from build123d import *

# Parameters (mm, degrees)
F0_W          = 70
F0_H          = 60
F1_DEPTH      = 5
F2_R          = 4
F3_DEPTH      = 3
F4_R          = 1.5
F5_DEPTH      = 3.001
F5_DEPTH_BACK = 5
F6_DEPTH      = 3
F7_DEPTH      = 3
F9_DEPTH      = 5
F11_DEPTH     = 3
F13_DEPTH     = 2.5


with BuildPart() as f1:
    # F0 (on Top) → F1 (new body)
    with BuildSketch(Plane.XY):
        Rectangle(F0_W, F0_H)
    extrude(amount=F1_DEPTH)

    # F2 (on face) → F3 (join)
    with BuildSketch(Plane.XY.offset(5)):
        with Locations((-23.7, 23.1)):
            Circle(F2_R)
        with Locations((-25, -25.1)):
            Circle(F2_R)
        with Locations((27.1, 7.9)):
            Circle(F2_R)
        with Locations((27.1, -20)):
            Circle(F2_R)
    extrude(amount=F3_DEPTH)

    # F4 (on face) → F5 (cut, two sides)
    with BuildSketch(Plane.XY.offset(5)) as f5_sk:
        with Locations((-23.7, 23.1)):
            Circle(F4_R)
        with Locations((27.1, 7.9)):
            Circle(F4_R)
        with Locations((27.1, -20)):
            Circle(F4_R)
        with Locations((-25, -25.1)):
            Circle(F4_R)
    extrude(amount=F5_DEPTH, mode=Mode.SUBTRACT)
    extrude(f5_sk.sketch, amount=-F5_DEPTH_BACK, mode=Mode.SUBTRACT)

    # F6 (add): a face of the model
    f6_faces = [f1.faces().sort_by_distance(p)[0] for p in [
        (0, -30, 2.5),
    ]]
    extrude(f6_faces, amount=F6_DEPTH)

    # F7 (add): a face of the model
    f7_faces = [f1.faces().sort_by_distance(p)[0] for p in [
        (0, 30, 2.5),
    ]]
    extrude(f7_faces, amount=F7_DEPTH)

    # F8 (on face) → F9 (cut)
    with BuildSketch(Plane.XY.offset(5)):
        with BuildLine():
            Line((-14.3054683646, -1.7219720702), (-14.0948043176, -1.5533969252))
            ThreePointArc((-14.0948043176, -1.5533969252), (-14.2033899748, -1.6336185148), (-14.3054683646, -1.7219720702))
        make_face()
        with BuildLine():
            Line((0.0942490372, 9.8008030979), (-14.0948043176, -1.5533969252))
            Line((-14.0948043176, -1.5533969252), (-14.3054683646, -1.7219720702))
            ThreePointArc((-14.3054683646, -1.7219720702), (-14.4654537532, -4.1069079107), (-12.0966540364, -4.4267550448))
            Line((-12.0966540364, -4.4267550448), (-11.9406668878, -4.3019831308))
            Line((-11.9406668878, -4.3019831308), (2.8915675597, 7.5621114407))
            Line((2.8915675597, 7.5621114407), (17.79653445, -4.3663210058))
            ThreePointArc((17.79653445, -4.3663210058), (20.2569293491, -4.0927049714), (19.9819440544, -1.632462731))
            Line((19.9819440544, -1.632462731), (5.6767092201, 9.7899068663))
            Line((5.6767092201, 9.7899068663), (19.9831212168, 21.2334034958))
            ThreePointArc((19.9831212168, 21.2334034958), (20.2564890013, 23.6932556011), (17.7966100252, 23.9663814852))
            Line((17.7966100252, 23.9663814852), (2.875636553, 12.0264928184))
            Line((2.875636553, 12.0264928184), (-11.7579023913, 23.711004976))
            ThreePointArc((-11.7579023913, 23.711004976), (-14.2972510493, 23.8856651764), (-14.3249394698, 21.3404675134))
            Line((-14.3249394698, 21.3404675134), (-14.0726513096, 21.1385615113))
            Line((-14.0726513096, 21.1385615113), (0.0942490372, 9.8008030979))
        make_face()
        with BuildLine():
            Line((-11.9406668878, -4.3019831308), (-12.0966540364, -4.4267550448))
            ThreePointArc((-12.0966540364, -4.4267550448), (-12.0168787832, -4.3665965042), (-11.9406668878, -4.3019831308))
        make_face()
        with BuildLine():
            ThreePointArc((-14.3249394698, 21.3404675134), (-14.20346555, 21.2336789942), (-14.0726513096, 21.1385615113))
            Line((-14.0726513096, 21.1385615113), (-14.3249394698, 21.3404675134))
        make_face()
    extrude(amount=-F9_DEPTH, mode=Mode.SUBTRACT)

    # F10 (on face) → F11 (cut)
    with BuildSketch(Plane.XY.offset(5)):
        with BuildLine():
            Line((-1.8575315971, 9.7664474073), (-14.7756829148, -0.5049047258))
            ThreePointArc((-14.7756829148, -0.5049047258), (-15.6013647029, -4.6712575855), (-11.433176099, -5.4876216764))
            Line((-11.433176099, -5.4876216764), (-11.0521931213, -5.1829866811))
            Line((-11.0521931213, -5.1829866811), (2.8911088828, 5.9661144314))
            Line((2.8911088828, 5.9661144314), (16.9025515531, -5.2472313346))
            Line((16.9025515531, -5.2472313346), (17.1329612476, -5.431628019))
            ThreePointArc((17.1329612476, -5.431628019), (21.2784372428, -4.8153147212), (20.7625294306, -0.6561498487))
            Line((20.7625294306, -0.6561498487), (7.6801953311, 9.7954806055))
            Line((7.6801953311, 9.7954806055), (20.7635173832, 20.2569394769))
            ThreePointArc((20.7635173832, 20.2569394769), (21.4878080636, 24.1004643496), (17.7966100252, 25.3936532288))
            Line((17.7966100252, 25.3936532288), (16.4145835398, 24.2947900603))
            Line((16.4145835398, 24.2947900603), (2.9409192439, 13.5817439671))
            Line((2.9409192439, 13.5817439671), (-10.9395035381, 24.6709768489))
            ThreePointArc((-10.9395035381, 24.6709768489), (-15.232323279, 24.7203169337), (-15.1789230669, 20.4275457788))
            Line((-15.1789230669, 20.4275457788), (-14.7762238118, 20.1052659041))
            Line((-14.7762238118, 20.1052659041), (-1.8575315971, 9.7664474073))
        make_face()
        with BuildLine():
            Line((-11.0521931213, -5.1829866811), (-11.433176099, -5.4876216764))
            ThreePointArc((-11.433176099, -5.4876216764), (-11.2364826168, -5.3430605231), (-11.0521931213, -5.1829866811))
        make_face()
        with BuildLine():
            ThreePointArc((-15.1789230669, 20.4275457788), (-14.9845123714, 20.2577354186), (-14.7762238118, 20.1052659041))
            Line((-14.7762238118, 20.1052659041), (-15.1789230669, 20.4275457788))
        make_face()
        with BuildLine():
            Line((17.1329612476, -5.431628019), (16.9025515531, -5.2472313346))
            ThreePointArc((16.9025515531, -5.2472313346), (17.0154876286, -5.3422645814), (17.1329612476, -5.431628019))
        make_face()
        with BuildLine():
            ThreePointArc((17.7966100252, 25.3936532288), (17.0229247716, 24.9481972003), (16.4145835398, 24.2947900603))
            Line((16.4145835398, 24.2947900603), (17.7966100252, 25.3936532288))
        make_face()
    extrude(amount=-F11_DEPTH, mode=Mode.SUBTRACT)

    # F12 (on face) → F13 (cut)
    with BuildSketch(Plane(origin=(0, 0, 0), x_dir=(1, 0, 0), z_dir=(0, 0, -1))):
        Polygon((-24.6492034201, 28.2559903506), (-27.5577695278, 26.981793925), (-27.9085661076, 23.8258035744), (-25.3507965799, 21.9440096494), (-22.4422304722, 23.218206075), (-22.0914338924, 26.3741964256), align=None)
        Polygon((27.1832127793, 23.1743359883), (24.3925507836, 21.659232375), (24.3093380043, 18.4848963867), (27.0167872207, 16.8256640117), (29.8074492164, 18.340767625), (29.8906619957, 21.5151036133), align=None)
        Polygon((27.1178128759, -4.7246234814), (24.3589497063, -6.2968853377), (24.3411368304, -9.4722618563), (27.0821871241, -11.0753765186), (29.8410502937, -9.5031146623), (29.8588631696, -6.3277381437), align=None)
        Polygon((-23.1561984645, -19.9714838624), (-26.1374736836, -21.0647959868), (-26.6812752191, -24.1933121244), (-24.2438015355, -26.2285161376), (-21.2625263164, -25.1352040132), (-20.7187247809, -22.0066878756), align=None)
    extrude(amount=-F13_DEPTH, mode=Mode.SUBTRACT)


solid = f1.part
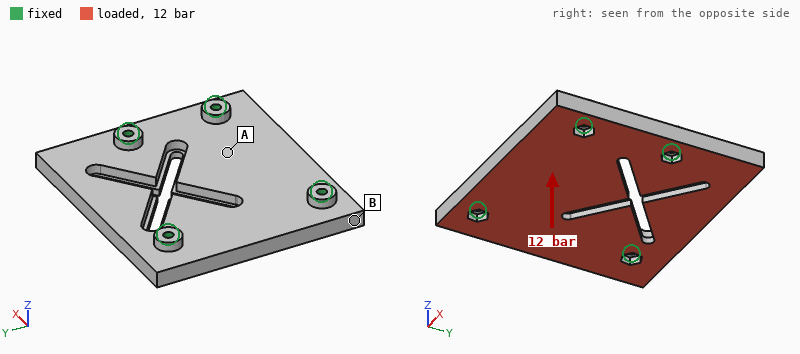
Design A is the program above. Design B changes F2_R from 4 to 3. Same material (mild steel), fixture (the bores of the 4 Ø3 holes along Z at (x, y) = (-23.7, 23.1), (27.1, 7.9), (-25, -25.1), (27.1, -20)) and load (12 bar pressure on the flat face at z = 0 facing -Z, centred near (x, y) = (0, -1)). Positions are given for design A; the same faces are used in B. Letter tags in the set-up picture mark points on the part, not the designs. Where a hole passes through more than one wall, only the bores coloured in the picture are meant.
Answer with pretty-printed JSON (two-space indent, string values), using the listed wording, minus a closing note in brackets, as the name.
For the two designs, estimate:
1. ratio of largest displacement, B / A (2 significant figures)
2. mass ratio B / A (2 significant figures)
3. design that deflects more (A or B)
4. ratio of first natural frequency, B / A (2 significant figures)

{
  "ratio of largest displacement, B / A": "1.1",
  "mass ratio B / A": "0.99",
  "design that deflects more": "B",
  "ratio of first natural frequency, B / A": "0.93"
}
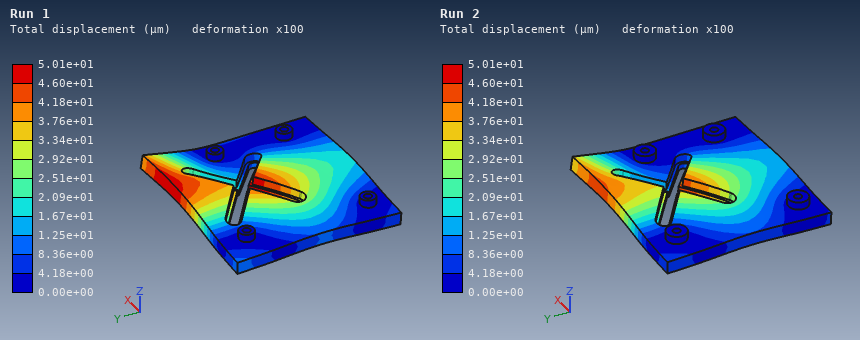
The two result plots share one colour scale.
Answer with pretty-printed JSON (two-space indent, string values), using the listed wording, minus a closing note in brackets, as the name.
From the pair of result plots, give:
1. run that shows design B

{
  "run that shows design B": "Run 1"
}
